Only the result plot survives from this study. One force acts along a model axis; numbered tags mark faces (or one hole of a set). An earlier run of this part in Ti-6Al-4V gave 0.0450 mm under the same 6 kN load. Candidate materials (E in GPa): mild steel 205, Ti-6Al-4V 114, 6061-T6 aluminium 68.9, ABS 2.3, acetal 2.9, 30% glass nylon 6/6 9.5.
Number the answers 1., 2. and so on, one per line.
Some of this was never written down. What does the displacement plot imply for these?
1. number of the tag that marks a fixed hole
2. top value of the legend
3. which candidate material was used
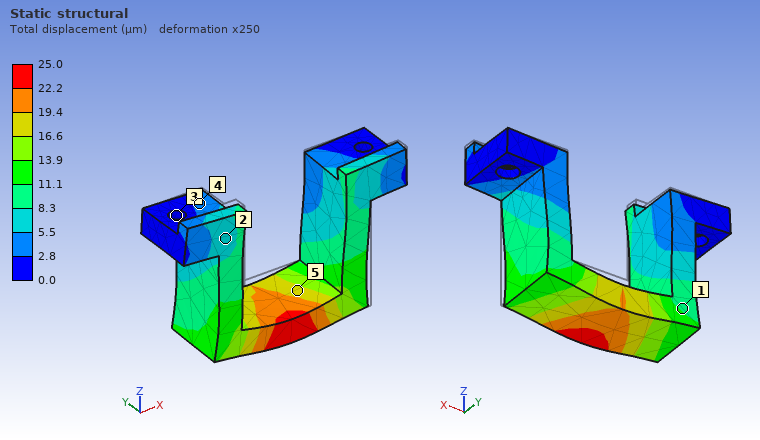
1. 3
2. 25.0 µm
3. mild steel
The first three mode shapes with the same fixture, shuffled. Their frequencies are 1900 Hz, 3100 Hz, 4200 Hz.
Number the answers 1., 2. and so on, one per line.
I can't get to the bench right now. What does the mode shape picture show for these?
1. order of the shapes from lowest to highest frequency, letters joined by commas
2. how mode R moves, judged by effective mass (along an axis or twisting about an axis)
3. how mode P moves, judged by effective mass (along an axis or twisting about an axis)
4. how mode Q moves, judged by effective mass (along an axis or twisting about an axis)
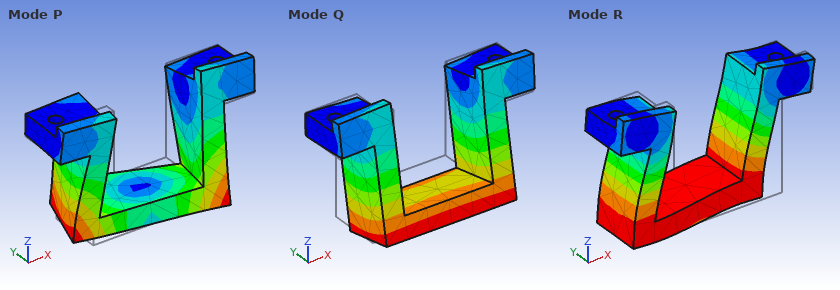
1. Q, R, P
2. along X
3. twisting about Z
4. along Y
